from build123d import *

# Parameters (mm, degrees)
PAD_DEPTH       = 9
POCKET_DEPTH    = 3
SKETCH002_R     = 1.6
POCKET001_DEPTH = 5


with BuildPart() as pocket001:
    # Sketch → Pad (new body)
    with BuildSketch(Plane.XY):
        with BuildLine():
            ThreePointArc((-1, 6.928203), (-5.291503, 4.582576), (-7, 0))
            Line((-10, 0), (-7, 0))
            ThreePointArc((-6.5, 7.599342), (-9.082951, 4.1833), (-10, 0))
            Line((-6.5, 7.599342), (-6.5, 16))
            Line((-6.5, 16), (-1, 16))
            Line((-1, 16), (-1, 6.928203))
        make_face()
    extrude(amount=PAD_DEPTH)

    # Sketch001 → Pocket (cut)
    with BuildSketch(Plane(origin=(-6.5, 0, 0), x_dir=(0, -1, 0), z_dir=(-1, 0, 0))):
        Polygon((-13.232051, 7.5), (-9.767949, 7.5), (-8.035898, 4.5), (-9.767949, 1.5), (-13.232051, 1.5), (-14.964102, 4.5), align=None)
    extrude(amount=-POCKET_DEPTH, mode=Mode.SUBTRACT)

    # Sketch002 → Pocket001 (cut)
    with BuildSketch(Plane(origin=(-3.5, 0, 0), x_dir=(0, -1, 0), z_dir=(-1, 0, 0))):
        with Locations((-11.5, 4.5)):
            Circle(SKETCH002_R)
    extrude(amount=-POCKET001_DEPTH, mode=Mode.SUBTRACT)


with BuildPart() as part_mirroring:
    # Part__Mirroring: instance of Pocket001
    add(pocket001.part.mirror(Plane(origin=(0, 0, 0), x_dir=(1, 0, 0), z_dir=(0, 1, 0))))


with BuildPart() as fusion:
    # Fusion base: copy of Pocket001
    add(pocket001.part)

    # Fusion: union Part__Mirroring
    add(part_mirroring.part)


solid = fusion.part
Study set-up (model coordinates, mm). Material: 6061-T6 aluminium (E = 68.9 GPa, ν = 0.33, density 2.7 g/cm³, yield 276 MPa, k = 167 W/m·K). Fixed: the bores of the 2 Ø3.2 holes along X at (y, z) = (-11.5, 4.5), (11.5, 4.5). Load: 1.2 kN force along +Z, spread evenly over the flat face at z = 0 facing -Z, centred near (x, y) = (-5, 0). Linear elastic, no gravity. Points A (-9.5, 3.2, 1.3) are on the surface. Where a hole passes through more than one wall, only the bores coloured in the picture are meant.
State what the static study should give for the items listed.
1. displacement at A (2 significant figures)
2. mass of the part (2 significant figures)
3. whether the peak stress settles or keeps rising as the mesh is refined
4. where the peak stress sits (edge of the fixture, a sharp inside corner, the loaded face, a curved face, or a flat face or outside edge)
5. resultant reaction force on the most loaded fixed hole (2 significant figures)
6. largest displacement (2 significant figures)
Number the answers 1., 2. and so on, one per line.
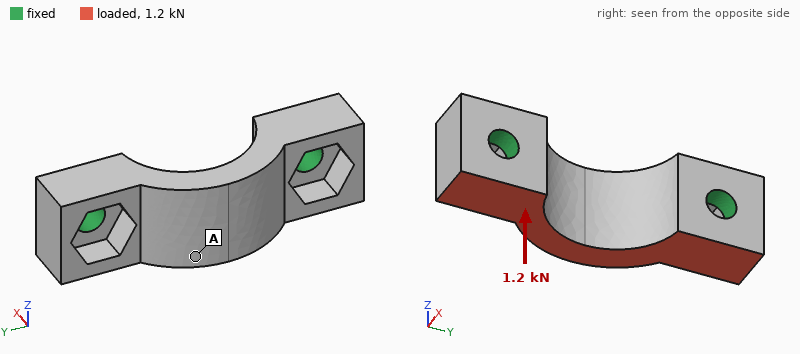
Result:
1. 21 µm
2. 3.0 g
3. keeps rising
4. edge of the fixture
5. 600 N
6. 24 µm
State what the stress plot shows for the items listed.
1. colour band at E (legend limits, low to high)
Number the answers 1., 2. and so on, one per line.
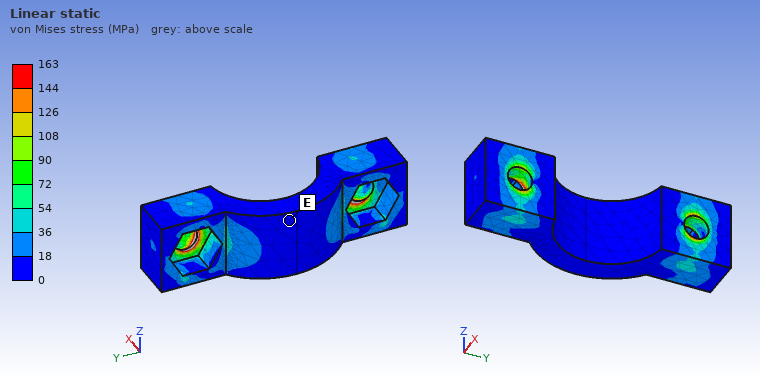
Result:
1. 0 to 18 MPa
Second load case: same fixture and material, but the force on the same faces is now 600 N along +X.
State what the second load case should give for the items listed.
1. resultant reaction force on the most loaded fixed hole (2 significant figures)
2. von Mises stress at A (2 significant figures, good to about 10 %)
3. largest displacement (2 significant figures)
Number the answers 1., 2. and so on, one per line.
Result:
1. 310 N
2. 14 MPa
3. 15 µm
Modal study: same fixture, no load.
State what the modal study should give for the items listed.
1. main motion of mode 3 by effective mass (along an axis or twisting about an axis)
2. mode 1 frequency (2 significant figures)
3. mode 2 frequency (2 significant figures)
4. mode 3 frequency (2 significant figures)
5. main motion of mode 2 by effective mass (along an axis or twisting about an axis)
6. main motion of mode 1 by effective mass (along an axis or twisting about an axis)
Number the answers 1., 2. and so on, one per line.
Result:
1. along X
2. 23 kHz
3. 44 kHz
4. 48 kHz
5. along Y
6. along Z
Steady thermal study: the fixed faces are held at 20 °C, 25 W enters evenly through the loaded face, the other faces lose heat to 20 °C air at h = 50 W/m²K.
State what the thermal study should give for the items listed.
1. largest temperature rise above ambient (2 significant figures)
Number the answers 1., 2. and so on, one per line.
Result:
1. 14 K
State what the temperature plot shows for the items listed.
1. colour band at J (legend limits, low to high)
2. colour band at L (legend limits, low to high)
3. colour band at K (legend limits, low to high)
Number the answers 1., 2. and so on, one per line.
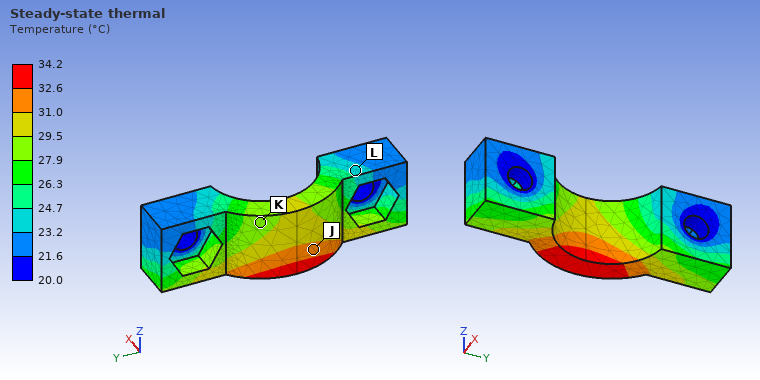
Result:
1. 31.0 to 32.6 °C
2. 23.2 to 24.7 °C
3. 27.9 to 29.5 °C
